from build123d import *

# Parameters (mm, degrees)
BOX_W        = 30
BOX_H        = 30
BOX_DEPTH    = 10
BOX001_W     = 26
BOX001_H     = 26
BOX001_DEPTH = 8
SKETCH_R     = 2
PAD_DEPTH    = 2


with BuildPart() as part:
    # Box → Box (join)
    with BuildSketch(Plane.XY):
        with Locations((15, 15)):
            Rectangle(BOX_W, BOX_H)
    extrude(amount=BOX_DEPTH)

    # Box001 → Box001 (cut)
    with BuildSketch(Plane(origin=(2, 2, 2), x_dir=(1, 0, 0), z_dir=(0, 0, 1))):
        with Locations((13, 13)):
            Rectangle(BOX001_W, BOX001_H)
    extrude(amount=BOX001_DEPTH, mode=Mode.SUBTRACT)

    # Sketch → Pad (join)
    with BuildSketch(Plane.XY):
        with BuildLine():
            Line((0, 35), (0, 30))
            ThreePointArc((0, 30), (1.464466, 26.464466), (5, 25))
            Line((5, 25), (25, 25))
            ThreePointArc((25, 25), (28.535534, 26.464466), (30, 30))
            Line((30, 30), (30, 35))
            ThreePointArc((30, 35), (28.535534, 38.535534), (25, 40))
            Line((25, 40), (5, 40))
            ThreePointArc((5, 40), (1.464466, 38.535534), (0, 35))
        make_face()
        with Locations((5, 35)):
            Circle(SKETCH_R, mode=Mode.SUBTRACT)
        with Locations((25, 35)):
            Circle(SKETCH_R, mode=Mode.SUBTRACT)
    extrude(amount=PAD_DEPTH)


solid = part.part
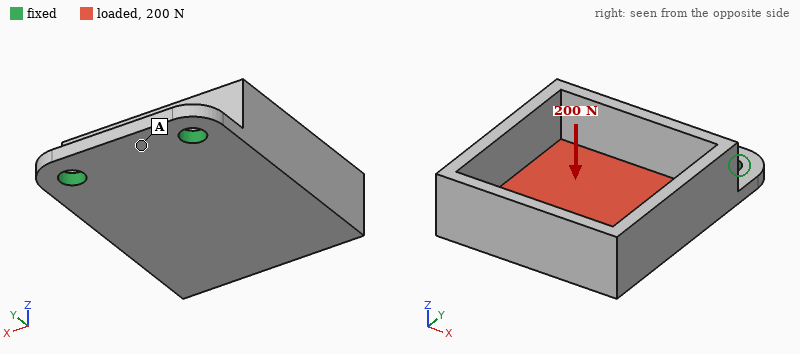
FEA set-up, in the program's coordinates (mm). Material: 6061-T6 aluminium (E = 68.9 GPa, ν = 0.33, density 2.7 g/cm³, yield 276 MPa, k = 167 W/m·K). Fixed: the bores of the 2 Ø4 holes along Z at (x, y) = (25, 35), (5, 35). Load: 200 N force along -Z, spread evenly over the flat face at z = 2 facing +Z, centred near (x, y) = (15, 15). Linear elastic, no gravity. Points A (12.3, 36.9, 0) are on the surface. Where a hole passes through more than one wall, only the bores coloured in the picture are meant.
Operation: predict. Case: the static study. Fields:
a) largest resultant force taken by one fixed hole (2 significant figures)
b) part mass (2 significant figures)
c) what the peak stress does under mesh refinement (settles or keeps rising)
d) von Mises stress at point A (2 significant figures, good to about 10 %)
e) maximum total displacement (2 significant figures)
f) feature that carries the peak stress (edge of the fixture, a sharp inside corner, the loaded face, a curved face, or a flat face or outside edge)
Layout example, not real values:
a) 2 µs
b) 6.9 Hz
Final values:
a) 110 N
b) 11 g
c) keeps rising
d) 33 MPa
e) 0.46 mm
f) edge of the fixture
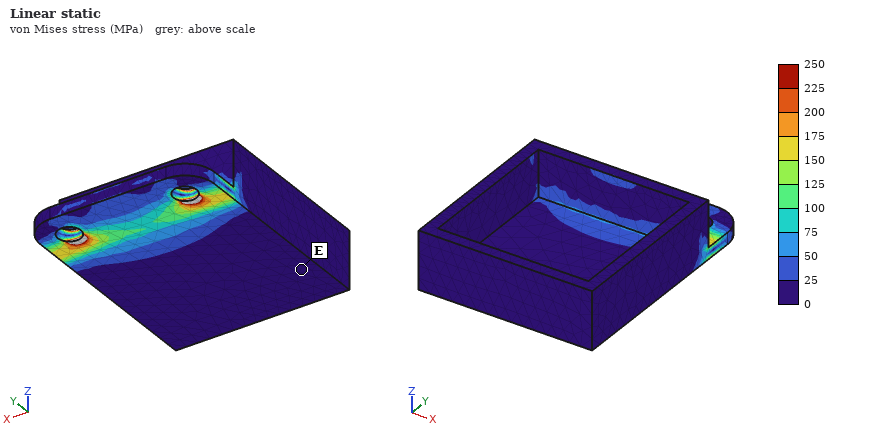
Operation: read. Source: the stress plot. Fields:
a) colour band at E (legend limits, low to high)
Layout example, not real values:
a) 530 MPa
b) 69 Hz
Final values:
a) 0 to 25 MPa
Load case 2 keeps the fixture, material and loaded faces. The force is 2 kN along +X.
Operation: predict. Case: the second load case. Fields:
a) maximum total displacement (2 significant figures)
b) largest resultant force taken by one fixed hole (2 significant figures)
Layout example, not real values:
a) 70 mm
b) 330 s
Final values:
a) 0.14 mm
b) 2.0 kN
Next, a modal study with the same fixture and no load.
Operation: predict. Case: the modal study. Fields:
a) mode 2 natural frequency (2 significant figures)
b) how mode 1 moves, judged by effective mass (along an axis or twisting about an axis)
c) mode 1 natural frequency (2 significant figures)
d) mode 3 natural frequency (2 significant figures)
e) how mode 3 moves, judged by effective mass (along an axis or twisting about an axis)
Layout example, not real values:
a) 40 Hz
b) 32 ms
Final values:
a) 3200 Hz
b) along Z
c) 1200 Hz
d) 9500 Hz
e) along X
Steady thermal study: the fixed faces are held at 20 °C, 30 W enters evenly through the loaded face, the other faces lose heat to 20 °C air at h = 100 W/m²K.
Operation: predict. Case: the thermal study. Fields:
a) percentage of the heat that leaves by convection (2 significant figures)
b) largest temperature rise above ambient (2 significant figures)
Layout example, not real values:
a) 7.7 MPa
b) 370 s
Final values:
a) 27 %
b) 35 K
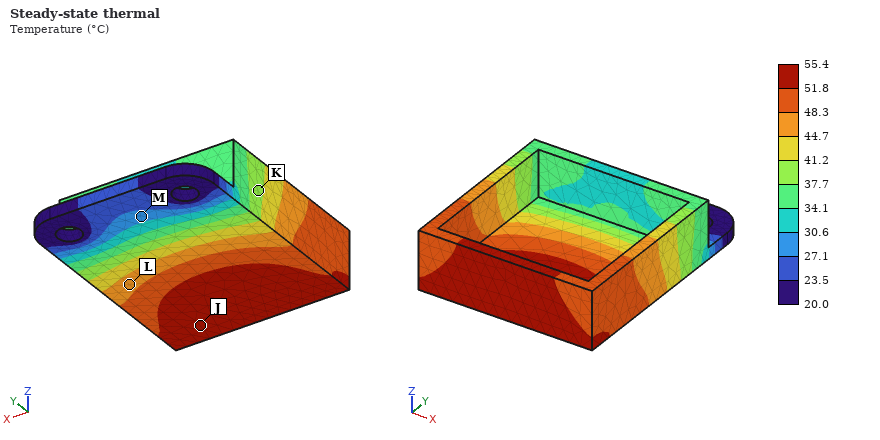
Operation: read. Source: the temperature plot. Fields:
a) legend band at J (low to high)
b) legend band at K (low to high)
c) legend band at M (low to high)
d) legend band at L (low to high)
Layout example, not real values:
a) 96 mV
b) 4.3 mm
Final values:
a) 51.8 to 55.4 °C
b) 37.7 to 41.2 °C
c) 27.1 to 30.6 °C
d) 44.7 to 48.3 °C
